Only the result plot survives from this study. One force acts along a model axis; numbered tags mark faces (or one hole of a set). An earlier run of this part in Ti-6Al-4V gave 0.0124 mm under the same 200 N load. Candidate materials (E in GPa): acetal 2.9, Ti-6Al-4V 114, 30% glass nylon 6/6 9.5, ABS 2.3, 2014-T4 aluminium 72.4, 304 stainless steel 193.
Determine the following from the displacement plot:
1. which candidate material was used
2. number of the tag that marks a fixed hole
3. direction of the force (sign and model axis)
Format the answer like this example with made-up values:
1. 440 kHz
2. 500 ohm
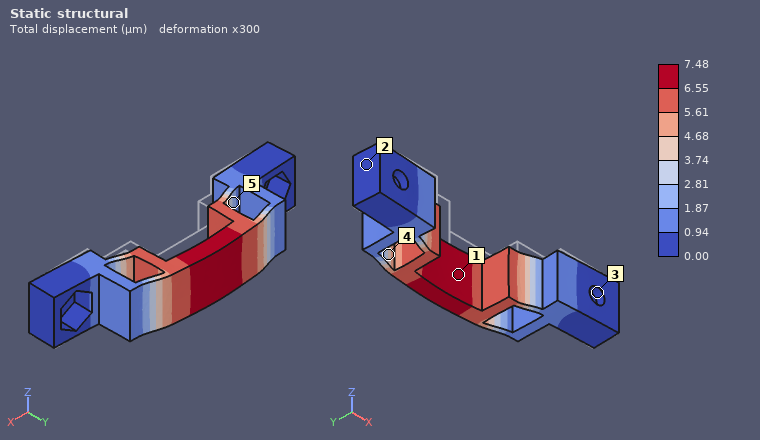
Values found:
1. 304 stainless steel
2. 3
3. +Y
